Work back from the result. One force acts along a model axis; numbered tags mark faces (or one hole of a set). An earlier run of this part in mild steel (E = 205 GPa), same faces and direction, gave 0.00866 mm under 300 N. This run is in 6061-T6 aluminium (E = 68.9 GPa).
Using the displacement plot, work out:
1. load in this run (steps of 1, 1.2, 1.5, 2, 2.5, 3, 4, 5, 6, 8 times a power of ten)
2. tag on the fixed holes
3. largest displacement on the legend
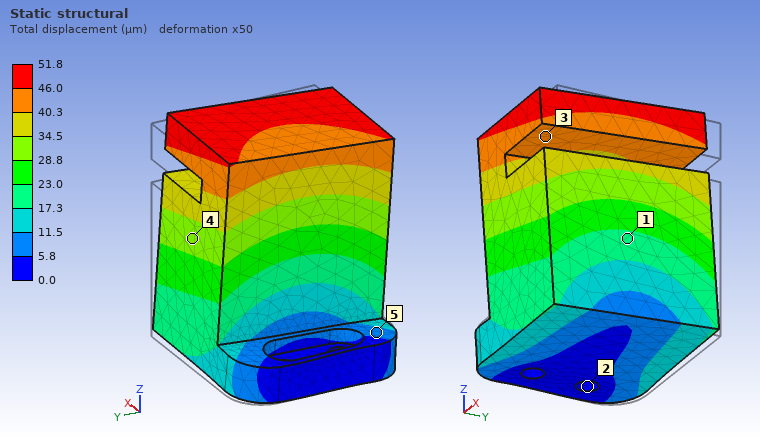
600 N
2
51.8 µm
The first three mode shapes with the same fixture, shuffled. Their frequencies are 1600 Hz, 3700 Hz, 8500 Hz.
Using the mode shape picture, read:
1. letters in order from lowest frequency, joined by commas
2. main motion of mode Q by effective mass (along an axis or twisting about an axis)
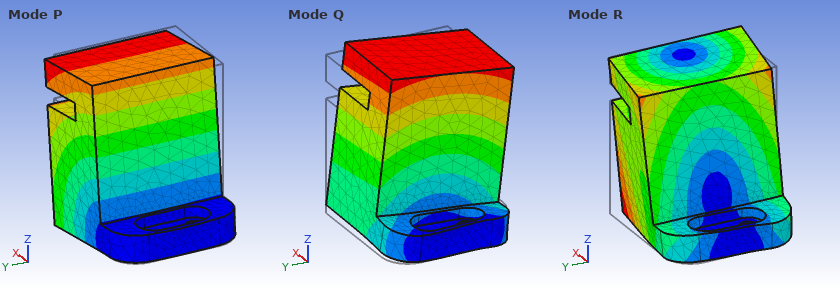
P, Q, R
along Y
